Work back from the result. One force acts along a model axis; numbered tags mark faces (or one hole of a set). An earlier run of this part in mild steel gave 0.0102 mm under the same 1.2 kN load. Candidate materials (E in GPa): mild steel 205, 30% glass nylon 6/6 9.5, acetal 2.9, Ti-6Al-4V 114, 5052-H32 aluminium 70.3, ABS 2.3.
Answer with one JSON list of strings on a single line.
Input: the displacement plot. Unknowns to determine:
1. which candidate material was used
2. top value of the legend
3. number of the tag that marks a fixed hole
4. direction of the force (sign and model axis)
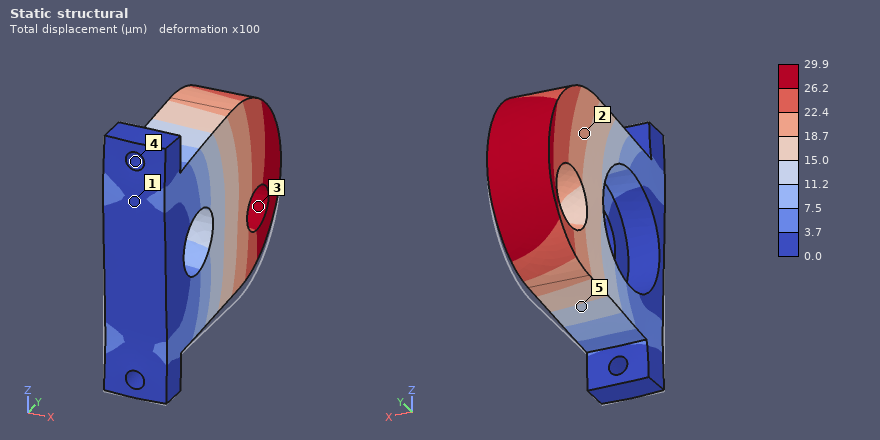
["5052-H32 aluminium", "29.9 µm", "4", "+Z"]
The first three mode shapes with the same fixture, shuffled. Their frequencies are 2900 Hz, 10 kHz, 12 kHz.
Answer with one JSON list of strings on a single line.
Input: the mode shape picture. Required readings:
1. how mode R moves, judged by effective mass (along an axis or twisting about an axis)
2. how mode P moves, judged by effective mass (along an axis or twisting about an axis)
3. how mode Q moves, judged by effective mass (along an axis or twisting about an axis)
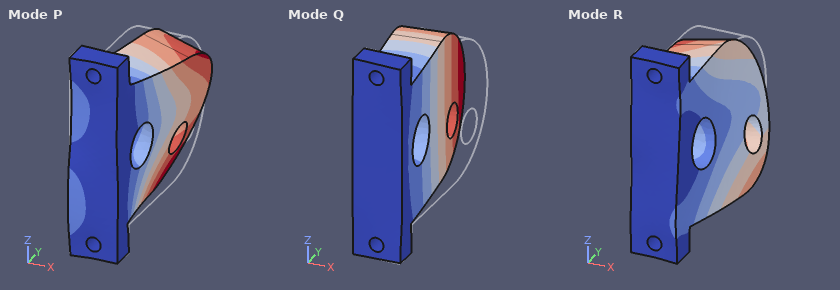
["along Z", "along Z", "along X"]
